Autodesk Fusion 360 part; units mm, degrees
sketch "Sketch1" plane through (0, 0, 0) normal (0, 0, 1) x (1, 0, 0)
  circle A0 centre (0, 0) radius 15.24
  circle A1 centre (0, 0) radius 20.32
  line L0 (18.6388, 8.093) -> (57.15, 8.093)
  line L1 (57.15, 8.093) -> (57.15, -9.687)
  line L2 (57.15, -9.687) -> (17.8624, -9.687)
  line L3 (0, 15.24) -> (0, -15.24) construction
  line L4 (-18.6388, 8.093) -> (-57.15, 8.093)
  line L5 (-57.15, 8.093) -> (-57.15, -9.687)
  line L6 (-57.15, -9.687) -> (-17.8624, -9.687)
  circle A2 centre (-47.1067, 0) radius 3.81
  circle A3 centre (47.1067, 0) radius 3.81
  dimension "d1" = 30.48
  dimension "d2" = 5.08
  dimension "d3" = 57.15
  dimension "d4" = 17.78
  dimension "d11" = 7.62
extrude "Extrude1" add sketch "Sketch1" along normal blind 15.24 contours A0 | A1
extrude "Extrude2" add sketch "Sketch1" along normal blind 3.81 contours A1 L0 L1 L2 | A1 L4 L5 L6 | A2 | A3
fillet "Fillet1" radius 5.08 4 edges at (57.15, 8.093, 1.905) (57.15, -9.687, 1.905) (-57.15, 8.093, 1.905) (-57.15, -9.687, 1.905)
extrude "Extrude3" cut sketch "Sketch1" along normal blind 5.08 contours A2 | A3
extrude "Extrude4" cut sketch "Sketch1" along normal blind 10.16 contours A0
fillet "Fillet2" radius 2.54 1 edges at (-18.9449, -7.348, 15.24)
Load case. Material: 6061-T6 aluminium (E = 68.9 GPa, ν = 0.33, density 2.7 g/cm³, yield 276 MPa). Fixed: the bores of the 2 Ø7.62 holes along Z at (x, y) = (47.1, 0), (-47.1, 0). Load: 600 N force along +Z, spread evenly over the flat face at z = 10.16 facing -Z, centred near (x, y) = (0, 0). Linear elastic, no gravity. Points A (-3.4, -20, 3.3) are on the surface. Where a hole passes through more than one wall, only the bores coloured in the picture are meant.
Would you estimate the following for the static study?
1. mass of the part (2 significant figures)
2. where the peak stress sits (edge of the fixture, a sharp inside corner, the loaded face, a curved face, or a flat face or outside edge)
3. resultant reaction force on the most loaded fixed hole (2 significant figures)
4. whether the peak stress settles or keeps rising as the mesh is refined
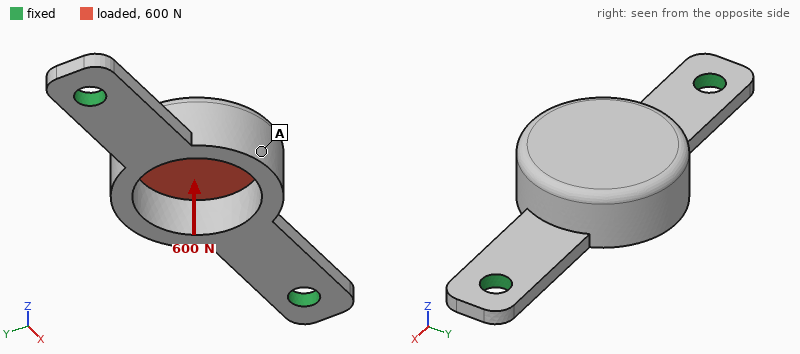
45 g
edge of the fixture
540 N
keeps rising
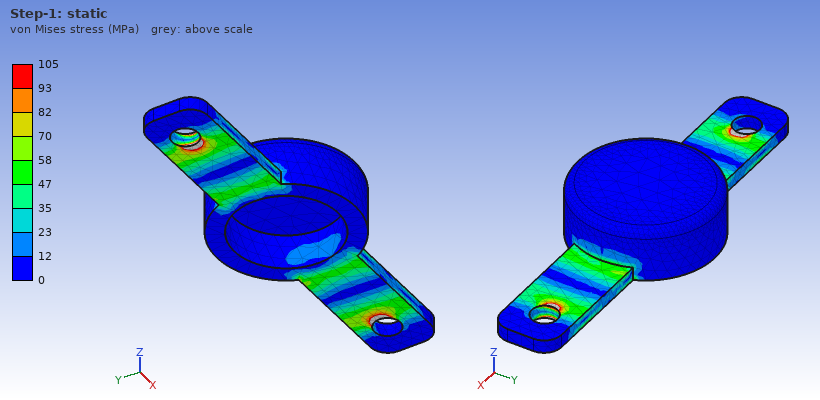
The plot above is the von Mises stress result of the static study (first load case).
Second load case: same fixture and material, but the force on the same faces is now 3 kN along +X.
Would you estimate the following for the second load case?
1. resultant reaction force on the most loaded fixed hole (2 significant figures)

1.5 kN
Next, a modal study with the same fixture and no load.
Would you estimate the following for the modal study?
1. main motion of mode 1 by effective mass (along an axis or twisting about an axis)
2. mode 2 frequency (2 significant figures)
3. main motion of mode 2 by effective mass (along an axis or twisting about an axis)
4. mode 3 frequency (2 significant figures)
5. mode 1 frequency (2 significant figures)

along Y
2100 Hz
along Z
4600 Hz
1600 Hz
